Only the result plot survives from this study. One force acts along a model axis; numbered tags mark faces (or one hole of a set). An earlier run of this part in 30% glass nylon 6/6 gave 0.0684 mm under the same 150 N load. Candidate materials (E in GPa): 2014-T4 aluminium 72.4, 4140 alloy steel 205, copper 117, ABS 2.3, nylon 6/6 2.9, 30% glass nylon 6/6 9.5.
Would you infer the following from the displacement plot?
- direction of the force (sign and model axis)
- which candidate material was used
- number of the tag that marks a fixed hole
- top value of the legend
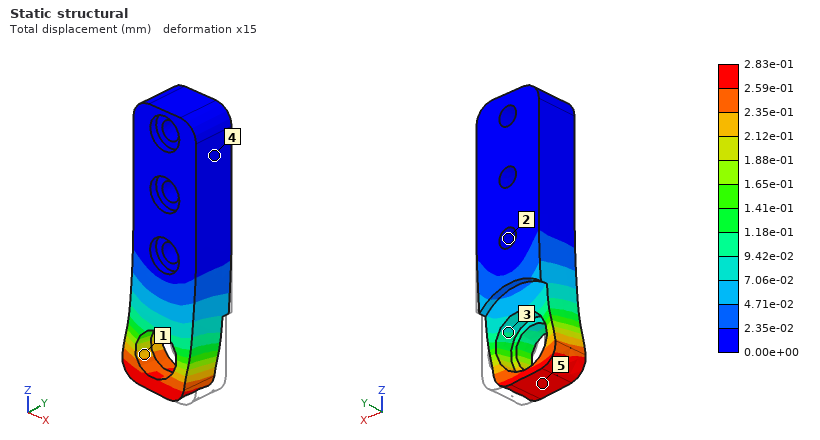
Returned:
-X
ABS
2
2.83e-01 mm
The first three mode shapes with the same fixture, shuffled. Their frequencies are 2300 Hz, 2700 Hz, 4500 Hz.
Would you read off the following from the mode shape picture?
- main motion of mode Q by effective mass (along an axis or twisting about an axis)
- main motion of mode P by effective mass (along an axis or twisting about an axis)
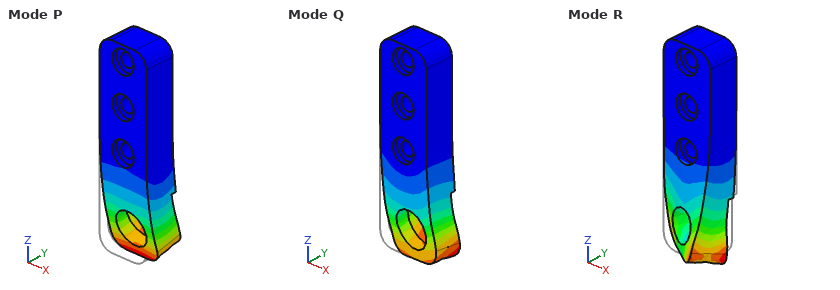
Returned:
along X
along Y
